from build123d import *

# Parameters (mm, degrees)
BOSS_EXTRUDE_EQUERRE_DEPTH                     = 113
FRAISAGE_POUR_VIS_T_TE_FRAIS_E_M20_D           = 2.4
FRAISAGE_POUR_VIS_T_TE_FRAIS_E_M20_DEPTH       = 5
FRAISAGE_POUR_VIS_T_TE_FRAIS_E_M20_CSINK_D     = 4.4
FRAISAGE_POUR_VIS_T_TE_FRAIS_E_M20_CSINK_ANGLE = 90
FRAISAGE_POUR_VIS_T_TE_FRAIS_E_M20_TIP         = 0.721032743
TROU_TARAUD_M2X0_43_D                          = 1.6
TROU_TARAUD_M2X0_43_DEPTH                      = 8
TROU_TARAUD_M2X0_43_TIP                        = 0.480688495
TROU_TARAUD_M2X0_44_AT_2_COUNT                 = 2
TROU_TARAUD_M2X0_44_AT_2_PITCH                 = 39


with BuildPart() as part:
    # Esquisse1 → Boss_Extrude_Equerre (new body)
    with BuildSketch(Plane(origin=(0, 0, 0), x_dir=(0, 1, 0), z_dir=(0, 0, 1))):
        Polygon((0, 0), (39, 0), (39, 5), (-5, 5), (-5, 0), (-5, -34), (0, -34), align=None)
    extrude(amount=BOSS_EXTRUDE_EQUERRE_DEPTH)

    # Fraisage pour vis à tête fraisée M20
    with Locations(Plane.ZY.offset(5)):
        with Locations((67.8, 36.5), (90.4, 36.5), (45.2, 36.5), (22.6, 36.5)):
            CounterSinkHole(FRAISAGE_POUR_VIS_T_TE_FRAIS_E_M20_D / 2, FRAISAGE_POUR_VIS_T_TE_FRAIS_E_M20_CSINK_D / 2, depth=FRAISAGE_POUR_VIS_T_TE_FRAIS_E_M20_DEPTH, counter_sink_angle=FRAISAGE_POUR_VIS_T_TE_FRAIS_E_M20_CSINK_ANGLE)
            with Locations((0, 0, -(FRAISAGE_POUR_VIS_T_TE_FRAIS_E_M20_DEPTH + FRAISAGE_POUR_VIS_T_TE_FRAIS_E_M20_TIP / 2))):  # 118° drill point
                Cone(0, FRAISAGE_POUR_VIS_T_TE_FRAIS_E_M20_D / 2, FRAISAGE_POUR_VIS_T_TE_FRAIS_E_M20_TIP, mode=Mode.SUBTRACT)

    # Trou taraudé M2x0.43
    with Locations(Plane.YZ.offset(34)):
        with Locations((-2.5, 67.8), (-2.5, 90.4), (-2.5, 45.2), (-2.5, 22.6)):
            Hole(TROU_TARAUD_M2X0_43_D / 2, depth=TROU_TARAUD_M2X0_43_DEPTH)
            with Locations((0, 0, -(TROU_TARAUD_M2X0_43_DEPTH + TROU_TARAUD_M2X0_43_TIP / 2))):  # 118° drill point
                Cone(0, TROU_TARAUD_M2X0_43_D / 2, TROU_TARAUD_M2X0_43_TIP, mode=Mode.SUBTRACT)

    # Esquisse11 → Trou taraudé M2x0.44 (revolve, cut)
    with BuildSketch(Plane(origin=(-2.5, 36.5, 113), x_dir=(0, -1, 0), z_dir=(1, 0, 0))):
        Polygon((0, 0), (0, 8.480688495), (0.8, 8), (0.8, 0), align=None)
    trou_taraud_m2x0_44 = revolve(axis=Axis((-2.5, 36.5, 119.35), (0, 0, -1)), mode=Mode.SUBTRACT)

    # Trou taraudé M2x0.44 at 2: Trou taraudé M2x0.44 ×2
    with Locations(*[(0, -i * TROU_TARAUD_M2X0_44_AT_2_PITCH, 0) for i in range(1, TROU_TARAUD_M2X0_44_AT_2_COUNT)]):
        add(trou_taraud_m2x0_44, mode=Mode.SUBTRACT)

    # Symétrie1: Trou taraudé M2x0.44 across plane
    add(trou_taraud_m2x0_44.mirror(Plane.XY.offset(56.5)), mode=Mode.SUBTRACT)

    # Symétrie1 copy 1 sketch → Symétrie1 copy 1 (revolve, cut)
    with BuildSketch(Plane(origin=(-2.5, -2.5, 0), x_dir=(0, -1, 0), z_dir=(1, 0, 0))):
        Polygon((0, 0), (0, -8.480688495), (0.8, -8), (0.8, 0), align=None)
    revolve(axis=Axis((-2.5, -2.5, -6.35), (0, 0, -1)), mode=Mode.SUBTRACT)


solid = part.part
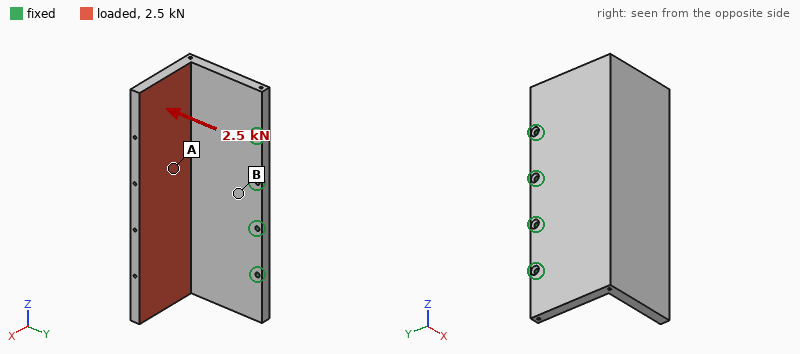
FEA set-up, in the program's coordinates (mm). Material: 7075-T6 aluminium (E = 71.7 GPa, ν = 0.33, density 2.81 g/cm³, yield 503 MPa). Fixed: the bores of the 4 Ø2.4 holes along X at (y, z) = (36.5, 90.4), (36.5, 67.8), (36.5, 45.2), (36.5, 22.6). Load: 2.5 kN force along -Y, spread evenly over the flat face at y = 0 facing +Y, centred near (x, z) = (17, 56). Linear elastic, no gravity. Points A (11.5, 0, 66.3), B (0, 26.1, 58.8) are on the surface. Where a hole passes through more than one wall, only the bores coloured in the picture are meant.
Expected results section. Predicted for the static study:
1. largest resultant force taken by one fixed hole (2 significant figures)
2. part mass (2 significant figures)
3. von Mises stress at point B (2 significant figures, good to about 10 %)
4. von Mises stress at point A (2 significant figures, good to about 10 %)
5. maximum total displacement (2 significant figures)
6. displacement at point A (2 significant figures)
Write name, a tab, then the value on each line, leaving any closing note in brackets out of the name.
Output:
largest resultant force taken by one fixed hole	700 N
part mass	120 g
von Mises stress at point B	100 MPa
von Mises stress at point A	37 MPa
maximum total displacement	1.3 mm
displacement at point A	0.69 mm
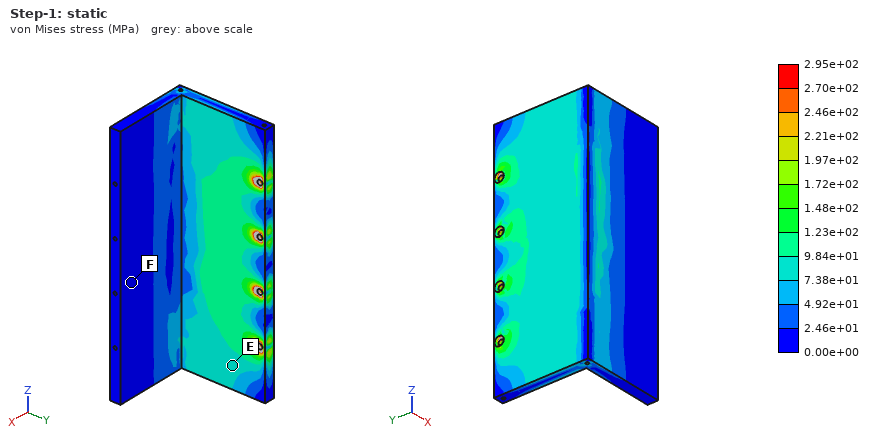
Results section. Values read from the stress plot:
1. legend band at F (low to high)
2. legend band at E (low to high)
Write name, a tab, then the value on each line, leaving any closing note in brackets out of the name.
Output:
legend band at F	0.00e+00 to 2.46e+01 MPa
legend band at E	7.38e+01 to 9.84e+01 MPa
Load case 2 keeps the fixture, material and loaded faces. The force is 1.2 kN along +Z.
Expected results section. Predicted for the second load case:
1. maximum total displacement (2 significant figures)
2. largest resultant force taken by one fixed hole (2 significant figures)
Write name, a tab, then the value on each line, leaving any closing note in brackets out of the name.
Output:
maximum total displacement	0.27 mm
largest resultant force taken by one fixed hole	710 N
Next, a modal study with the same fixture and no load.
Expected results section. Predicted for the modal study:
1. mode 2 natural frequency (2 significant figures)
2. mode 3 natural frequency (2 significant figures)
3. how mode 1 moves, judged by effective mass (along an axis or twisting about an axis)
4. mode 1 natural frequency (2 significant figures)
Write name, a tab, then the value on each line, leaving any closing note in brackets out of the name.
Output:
mode 2 natural frequency	1200 Hz
mode 3 natural frequency	2500 Hz
how mode 1 moves, judged by effective mass	along X
mode 1 natural frequency	770 Hz
